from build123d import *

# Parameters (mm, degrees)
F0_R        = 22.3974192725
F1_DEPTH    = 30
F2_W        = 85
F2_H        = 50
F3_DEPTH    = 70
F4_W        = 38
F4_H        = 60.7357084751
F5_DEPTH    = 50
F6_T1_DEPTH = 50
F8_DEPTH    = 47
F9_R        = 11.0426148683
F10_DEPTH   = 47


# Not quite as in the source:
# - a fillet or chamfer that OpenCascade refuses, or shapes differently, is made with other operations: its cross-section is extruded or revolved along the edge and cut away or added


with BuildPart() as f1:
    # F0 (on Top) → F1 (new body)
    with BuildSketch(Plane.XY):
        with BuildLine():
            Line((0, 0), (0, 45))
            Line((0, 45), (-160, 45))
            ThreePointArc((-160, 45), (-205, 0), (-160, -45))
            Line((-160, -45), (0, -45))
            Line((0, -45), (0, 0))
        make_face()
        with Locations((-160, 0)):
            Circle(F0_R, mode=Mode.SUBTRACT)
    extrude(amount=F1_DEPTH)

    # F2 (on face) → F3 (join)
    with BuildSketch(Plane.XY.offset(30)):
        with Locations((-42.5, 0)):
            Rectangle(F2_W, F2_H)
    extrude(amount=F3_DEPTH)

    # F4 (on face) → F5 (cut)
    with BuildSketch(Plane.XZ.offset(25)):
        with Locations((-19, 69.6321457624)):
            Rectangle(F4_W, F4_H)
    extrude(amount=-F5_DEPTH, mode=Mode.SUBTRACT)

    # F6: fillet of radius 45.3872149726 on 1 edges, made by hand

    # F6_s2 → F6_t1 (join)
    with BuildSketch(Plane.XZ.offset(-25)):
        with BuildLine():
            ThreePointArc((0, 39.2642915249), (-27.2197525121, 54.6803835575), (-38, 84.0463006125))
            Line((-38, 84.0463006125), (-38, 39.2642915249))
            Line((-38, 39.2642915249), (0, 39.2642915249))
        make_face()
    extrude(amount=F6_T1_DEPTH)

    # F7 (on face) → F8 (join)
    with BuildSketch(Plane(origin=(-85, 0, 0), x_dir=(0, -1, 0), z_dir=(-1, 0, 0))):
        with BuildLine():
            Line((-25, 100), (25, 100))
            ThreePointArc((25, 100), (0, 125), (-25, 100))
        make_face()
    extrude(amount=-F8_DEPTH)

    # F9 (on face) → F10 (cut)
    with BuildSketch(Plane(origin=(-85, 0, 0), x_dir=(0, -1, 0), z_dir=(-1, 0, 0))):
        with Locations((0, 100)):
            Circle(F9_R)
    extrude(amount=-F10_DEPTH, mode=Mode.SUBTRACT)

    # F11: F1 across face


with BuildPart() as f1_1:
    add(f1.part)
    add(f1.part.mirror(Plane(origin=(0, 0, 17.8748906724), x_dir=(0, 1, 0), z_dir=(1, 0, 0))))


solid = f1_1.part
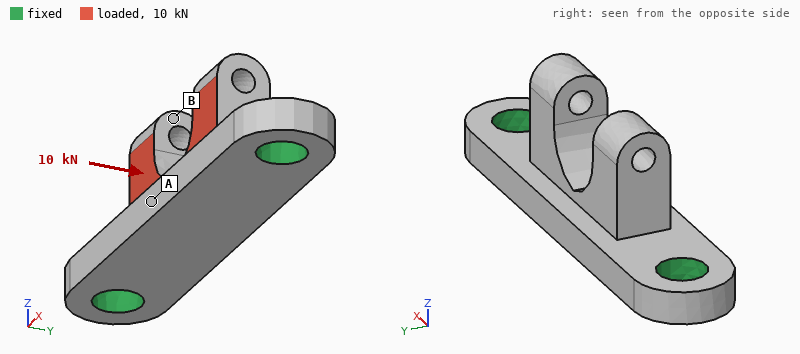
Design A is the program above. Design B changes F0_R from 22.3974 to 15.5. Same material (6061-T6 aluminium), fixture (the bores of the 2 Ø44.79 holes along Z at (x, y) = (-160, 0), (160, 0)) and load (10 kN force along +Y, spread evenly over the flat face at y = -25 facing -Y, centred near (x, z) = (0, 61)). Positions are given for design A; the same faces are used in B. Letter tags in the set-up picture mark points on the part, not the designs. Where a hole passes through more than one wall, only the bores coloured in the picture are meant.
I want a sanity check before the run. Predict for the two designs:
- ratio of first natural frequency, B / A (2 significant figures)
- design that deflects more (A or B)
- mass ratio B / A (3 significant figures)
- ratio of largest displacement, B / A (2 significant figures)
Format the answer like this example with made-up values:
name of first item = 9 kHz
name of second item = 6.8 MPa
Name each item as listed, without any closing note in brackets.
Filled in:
ratio of first natural frequency, B / A = 0.91
design that deflects more = B
mass ratio B / A = 1.03
ratio of largest displacement, B / A = 1.2
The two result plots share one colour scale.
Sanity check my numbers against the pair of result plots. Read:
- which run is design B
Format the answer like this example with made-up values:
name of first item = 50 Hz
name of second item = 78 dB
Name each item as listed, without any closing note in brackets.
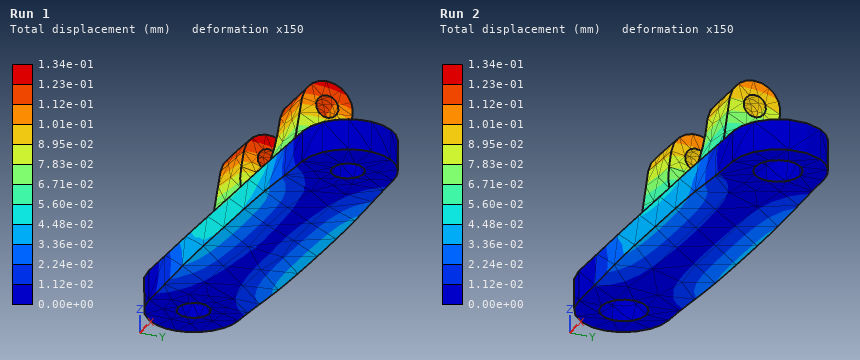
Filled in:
which run is design B = Run 1
